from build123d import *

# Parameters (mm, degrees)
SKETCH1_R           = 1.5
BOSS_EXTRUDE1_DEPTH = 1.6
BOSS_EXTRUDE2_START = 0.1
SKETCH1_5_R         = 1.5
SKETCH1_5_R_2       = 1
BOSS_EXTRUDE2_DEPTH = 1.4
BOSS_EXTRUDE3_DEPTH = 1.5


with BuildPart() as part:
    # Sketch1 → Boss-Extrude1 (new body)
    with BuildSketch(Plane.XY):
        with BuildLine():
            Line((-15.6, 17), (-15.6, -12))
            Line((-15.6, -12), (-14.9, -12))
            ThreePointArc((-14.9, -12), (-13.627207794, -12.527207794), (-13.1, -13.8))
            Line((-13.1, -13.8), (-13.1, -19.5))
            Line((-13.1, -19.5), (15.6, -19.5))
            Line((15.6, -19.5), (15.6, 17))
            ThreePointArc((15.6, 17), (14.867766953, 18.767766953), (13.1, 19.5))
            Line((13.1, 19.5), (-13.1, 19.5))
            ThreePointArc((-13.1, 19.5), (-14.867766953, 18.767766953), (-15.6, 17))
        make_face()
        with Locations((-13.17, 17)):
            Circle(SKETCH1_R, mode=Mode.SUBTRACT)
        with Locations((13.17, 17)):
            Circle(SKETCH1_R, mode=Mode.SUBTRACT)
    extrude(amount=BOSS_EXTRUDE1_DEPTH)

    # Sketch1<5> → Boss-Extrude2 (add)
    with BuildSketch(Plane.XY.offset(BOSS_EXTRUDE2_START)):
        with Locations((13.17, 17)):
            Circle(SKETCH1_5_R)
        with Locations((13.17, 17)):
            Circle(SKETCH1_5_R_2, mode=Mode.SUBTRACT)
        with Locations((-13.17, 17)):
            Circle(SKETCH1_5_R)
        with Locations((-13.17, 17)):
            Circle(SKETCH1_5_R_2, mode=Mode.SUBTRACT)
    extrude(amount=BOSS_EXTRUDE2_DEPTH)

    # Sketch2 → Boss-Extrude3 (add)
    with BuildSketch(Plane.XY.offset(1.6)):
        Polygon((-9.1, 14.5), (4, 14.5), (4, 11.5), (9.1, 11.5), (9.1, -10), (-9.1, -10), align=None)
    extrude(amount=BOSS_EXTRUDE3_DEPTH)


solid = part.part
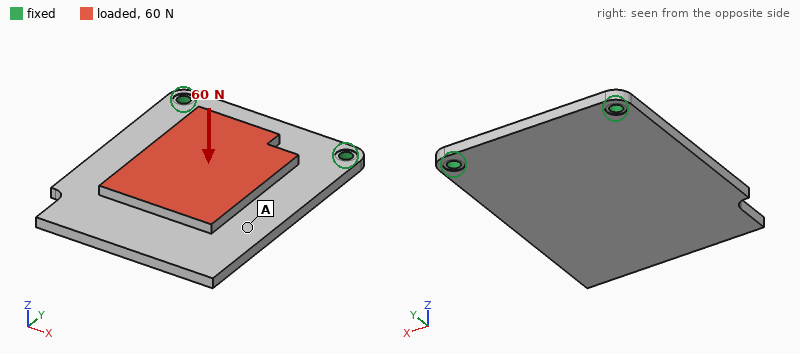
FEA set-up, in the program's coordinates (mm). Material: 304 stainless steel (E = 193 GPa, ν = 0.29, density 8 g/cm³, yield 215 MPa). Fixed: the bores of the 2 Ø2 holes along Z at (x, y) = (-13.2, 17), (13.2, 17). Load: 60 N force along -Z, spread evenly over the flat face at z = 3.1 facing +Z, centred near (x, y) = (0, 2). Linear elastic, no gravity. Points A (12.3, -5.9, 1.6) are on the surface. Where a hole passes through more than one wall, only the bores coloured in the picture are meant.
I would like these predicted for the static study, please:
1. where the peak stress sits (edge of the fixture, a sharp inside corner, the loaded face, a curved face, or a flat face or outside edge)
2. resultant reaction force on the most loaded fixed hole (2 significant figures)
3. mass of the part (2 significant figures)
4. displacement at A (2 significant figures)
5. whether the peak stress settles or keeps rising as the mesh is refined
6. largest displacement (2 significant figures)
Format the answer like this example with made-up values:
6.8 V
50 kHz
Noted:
edge of the fixture
31 N
20 g
0.074 mm
keeps rising
0.13 mm
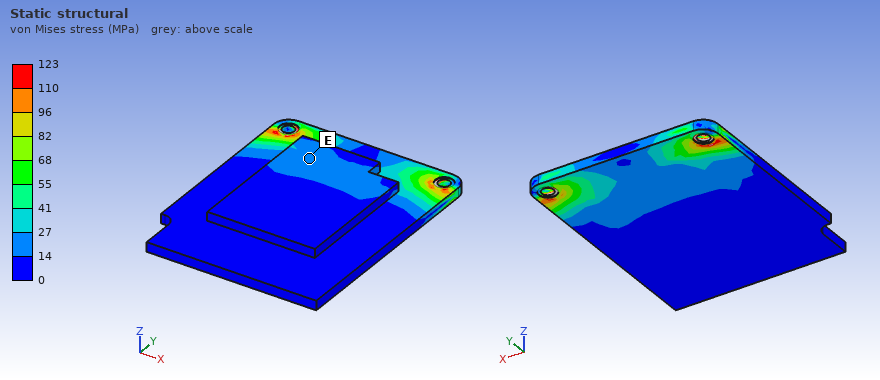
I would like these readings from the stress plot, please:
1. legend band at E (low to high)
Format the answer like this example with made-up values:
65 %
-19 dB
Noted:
14 to 27 MPa
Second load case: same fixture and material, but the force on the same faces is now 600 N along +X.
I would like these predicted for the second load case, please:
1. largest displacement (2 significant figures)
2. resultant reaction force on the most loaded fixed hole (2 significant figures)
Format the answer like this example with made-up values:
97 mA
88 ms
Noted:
18 µm
460 N
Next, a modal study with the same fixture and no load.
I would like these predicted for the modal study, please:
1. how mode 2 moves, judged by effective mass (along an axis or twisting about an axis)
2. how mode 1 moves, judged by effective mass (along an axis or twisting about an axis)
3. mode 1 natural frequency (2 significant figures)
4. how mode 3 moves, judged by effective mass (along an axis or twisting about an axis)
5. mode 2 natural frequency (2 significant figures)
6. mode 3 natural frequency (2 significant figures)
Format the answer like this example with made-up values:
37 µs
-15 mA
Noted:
twisting about Y
along Z
920 Hz
along Z
4400 Hz
7600 Hz
